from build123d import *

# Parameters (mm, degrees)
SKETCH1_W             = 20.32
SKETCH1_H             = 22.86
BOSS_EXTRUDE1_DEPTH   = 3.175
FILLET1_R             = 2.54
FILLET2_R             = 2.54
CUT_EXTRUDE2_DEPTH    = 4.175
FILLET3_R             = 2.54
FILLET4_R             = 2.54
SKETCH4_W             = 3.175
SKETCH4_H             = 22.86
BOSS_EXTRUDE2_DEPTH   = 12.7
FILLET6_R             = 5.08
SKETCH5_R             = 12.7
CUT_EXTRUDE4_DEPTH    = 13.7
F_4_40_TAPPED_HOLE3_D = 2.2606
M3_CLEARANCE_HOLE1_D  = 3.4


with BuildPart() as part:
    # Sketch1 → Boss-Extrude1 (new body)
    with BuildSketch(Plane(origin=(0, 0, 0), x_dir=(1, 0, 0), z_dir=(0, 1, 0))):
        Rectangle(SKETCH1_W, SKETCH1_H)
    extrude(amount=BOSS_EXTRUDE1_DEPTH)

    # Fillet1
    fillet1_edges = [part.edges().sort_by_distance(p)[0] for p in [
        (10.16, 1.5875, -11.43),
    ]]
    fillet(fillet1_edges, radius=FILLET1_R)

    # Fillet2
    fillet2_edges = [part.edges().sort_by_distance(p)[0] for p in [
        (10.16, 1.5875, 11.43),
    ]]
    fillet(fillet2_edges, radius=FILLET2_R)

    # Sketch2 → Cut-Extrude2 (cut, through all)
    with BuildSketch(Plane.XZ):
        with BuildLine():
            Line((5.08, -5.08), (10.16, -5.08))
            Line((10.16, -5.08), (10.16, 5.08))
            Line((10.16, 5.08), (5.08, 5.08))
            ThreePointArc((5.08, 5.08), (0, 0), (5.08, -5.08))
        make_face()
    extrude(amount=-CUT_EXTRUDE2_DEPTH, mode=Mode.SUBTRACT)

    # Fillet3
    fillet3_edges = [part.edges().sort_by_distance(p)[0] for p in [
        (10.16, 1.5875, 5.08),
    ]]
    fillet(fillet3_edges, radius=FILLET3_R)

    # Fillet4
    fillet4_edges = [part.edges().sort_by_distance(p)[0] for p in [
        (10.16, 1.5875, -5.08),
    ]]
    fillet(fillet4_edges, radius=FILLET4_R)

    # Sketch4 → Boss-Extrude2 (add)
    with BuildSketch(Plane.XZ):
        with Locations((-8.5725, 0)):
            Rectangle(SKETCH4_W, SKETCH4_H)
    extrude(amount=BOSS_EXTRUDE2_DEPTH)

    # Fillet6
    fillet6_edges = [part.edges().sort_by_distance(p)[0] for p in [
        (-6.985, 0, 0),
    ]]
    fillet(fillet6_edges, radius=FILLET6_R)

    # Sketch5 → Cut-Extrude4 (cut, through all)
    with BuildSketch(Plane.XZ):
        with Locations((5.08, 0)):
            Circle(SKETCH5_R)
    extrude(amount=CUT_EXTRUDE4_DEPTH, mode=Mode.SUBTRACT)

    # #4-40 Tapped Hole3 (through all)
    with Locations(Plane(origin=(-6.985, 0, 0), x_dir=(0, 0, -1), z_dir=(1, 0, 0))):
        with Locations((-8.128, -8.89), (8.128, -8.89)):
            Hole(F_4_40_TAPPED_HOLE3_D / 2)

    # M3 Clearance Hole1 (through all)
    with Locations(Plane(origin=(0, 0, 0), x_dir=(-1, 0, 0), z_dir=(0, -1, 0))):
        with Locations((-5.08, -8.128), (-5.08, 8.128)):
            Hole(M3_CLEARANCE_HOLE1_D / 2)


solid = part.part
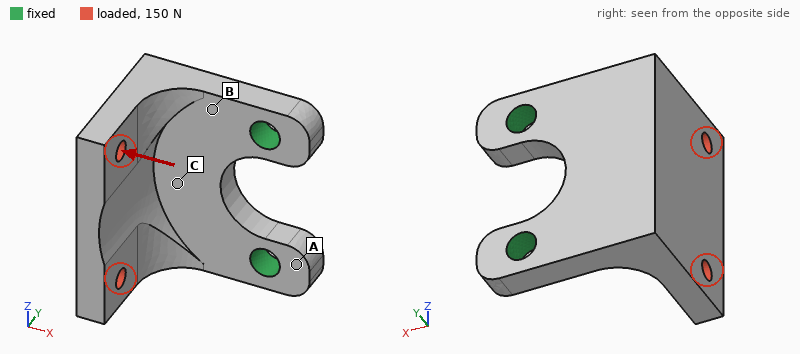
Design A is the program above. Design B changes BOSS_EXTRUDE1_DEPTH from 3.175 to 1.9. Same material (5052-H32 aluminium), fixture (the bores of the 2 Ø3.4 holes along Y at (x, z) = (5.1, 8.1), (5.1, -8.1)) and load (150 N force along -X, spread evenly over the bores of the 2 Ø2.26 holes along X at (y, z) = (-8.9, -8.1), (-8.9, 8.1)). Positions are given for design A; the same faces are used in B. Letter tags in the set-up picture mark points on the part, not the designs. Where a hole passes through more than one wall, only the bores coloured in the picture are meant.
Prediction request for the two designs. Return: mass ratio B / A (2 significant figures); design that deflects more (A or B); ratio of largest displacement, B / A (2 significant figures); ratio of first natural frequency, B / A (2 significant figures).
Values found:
0.78
B
3.5
0.52
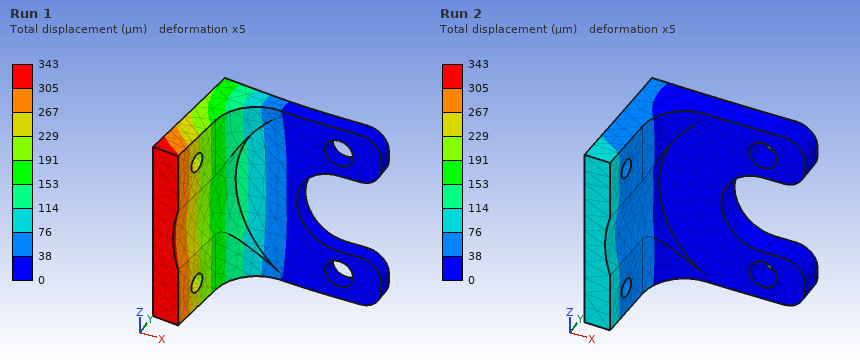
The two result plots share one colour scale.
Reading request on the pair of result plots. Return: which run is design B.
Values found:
Run 1
